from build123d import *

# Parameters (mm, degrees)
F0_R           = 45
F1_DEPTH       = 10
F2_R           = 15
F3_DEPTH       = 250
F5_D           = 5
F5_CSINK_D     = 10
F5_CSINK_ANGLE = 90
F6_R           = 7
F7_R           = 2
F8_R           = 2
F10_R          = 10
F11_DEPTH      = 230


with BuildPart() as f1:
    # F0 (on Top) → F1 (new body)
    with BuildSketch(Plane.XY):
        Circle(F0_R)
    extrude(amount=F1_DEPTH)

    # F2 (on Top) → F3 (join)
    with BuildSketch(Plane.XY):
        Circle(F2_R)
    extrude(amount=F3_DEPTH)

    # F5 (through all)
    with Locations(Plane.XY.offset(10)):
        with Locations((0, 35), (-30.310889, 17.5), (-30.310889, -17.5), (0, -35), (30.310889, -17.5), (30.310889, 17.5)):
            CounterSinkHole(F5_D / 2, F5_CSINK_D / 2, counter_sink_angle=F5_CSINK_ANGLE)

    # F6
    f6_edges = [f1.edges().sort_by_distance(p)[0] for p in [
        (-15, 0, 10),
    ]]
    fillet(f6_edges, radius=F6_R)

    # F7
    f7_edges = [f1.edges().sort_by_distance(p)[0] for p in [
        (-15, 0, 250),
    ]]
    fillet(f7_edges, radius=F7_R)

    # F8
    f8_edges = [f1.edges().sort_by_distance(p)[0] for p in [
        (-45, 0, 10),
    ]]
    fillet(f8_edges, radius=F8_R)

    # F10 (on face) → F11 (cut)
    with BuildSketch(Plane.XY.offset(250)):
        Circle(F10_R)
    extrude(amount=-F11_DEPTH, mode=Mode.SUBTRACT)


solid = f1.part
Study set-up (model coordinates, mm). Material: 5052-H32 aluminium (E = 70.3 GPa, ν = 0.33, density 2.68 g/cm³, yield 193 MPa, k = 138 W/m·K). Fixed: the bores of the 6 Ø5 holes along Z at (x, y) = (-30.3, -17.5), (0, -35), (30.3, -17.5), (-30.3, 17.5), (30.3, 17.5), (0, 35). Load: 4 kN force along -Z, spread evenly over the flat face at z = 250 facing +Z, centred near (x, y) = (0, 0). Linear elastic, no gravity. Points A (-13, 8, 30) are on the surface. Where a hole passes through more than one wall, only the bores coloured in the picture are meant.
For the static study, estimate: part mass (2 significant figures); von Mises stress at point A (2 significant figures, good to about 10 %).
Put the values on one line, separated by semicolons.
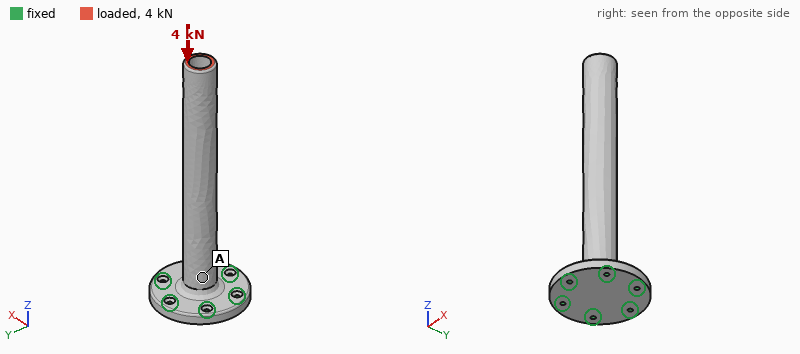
430 g; 9.6 MPa
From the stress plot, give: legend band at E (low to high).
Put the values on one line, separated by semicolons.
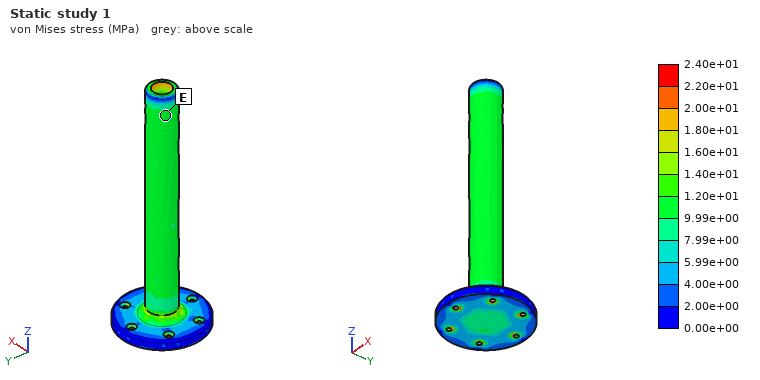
9.99e+00 to 1.20e+01 MPa
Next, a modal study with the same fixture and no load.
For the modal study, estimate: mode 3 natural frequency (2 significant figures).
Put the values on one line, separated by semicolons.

2400 Hz
